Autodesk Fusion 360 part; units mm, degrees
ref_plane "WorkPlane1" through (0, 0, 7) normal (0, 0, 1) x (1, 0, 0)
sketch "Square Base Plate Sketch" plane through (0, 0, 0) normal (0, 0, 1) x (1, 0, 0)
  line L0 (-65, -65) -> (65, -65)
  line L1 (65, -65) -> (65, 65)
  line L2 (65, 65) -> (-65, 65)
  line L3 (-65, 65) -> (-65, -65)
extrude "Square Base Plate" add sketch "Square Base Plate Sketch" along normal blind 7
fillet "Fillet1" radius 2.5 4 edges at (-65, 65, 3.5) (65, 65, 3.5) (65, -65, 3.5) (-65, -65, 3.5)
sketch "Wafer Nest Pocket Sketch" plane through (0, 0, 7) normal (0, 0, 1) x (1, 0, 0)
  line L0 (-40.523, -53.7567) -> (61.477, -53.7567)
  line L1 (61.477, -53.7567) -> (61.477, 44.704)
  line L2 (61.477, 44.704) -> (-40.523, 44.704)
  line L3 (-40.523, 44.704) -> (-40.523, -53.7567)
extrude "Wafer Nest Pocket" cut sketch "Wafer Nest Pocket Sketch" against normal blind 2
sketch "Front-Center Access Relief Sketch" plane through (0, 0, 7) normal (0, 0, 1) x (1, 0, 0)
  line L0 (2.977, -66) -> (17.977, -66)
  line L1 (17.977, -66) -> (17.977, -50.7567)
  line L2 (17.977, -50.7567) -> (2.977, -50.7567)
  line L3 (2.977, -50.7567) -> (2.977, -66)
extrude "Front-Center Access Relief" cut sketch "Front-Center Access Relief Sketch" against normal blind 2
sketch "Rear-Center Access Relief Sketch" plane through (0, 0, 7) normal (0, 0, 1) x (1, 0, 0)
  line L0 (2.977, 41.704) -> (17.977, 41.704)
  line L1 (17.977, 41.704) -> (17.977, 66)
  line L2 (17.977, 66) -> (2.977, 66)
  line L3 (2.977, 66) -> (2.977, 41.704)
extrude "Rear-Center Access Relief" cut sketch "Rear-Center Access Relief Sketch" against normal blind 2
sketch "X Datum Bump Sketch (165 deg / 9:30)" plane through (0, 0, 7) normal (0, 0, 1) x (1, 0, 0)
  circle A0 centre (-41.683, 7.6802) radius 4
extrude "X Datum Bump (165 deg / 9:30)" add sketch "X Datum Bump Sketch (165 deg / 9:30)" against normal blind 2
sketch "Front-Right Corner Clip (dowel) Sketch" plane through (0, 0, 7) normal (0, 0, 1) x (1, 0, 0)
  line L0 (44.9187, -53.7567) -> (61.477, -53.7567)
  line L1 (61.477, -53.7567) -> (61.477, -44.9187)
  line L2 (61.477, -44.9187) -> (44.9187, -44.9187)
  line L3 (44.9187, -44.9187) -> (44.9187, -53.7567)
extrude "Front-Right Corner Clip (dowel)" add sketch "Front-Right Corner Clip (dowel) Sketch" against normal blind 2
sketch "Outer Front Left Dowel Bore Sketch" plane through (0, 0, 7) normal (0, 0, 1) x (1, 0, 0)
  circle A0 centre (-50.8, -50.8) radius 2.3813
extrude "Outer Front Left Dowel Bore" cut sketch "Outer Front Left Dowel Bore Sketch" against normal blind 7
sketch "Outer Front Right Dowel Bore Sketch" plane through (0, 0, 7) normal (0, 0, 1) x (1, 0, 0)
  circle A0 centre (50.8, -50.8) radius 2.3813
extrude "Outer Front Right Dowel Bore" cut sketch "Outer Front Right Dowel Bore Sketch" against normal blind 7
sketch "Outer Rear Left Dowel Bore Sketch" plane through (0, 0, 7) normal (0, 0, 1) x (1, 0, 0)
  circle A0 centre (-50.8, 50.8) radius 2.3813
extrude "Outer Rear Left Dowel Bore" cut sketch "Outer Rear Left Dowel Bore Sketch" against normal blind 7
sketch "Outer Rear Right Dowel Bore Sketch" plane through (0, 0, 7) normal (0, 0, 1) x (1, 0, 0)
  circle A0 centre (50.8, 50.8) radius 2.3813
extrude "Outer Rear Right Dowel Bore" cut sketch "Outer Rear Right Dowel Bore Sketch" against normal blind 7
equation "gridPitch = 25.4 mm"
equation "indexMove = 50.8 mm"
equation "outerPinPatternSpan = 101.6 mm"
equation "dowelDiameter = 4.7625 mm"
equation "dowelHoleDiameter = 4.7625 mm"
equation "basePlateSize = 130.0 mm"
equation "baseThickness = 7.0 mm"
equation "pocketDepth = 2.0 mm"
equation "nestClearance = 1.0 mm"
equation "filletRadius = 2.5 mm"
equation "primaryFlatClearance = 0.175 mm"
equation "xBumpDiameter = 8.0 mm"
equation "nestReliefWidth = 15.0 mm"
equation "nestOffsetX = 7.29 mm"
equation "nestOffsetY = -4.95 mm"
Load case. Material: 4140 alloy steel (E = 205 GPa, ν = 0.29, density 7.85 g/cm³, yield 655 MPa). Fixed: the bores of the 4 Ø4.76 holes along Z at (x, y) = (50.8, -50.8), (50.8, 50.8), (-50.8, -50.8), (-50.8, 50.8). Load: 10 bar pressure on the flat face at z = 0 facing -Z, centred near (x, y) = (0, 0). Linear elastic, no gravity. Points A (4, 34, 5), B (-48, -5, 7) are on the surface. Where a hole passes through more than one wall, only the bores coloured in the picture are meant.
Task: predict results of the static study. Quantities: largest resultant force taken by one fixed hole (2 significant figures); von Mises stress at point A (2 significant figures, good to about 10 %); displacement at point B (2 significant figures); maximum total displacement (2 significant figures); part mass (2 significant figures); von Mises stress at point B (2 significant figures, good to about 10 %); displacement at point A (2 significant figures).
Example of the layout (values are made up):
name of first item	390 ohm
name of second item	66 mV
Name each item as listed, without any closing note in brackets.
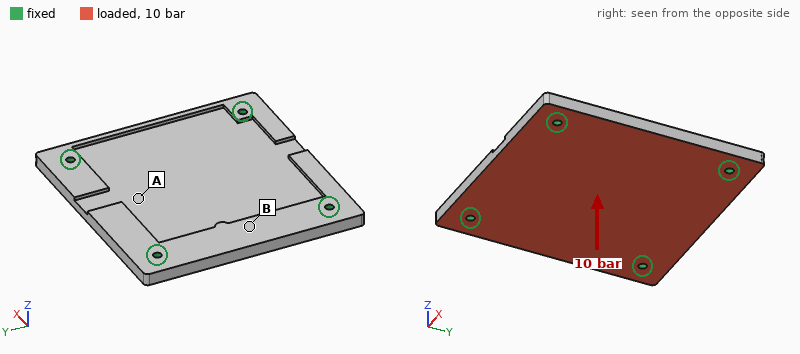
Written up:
largest resultant force taken by one fixed hole	4.9 kN
von Mises stress at point A	80 MPa
displacement at point B	0.10 mm
maximum total displacement	0.24 mm
part mass	760 g
von Mises stress at point B	100 MPa
displacement at point A	0.17 mm
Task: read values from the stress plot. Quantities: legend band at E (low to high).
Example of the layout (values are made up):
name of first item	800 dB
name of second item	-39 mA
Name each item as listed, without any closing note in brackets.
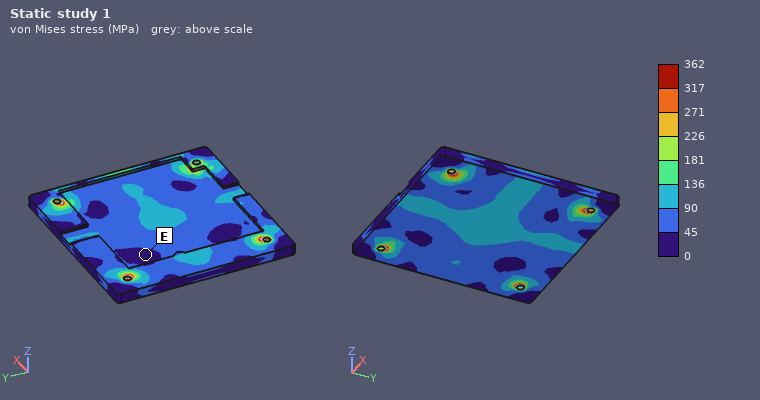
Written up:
legend band at E	0 to 45 MPa
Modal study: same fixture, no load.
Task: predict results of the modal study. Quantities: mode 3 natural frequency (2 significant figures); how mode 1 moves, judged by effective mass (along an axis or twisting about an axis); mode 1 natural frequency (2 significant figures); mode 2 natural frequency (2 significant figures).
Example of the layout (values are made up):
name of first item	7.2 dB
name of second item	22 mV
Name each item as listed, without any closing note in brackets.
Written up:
mode 3 natural frequency	3200 Hz
how mode 1 moves, judged by effective mass	along Z
mode 1 natural frequency	2000 Hz
mode 2 natural frequency	3100 Hz
